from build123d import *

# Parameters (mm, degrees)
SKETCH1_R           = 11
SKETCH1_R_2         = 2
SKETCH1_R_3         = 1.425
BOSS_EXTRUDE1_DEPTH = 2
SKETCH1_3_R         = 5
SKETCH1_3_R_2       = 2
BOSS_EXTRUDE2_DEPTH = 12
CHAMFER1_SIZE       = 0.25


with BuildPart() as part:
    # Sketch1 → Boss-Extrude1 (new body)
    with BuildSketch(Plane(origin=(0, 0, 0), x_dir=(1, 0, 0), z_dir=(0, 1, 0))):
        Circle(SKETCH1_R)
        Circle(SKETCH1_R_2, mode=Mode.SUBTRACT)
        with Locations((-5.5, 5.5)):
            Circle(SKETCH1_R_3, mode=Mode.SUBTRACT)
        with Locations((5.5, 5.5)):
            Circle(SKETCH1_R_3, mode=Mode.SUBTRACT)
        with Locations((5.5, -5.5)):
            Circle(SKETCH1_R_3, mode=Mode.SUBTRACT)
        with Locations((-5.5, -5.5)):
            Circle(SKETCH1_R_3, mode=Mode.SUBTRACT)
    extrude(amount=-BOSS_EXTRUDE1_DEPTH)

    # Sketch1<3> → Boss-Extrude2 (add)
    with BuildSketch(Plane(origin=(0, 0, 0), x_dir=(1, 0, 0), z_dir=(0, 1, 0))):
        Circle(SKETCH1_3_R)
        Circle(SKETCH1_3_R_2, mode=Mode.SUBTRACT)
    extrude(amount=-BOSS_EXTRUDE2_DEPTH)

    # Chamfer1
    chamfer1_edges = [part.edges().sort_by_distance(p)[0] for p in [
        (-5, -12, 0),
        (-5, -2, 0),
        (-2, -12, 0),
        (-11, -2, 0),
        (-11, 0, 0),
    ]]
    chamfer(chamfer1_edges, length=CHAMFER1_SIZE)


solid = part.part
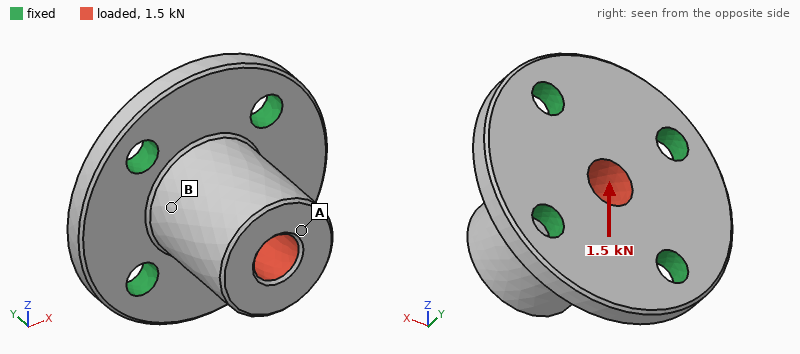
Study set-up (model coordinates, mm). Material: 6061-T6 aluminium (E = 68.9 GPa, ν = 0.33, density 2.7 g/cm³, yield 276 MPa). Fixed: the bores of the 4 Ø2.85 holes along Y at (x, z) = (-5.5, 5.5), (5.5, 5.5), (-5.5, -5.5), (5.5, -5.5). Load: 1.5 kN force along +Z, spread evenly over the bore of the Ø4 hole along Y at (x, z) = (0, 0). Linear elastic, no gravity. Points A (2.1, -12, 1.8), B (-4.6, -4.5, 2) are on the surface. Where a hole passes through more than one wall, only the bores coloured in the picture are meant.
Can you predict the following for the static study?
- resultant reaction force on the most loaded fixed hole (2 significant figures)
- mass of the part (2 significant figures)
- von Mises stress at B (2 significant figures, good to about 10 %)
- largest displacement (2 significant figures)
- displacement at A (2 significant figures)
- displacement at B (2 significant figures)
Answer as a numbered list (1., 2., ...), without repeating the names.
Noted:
1. 560 N
2. 3.6 g
3. 32 MPa
4. 26 µm
5. 24 µm
6. 8.2 µm
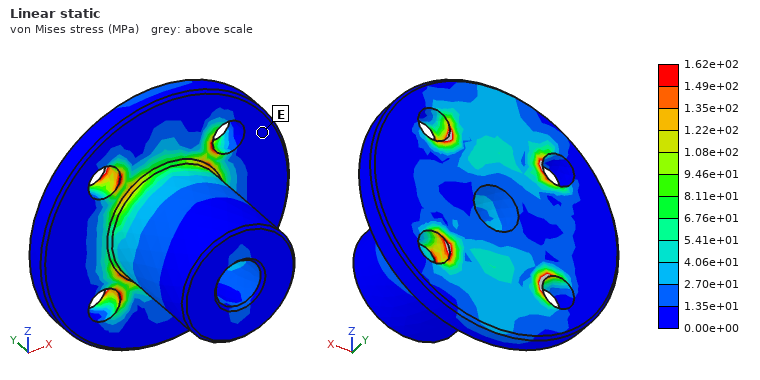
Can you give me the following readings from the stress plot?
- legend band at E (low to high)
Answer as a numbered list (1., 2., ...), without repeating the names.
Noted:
1. 0.00e+00 to 1.35e+01 MPa
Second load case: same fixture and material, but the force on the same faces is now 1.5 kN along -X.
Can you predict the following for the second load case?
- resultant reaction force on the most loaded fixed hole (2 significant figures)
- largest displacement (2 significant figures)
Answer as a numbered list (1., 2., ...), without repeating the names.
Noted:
1. 560 N
2. 26 µm
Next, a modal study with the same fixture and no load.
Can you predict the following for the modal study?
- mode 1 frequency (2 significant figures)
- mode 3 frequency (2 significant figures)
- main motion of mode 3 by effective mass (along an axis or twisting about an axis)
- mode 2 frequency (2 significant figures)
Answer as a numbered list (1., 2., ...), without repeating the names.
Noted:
1. 30 kHz
2. 51 kHz
3. along Y
4. 30 kHz
